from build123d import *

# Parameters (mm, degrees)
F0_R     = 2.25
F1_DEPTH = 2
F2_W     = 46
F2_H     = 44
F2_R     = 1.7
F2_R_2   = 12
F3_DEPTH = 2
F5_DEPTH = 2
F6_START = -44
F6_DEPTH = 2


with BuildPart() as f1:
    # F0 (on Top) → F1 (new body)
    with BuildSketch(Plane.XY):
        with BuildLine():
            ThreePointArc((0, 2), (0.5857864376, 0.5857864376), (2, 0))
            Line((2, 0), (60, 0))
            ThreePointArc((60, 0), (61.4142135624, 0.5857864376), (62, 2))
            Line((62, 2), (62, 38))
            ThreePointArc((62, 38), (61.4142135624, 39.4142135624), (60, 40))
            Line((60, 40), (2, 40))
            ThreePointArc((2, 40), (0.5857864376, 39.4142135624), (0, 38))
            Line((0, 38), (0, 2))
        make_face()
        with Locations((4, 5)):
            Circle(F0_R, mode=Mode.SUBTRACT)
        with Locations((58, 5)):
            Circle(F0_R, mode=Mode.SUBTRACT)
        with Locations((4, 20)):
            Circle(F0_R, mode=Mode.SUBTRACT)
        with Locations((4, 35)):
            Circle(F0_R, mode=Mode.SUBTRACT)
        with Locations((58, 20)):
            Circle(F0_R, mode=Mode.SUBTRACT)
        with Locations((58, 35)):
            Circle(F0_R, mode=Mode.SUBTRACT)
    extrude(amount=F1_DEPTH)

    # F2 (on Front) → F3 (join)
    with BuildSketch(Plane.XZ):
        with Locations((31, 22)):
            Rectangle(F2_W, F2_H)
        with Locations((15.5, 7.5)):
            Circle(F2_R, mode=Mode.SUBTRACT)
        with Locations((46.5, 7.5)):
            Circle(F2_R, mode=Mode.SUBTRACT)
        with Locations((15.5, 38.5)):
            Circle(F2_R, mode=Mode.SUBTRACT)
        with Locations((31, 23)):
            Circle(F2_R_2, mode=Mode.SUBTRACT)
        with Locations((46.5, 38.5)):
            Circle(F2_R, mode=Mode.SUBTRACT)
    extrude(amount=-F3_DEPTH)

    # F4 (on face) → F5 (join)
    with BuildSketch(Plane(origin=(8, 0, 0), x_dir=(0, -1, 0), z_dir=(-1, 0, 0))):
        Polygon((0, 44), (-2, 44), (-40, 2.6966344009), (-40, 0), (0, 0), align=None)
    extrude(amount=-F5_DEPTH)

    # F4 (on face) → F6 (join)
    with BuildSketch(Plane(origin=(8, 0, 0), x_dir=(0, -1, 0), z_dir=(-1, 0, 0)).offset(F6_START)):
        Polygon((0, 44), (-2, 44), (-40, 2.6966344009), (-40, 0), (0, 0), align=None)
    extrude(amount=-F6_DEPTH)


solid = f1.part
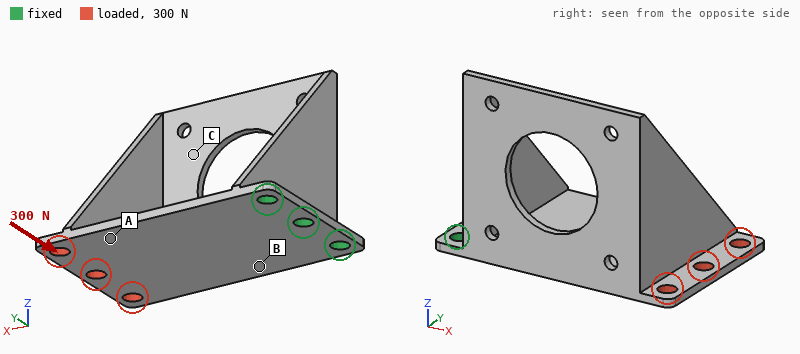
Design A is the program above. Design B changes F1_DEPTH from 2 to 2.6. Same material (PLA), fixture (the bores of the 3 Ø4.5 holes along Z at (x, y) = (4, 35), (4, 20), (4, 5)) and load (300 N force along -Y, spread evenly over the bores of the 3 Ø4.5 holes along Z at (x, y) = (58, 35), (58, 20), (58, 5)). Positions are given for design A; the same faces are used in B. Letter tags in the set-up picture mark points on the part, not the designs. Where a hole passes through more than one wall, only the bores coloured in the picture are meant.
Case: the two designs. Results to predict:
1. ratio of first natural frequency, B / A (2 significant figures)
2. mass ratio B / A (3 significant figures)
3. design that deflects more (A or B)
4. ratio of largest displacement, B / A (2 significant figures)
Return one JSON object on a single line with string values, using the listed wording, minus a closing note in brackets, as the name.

{"ratio of first natural frequency, B / A": "1.3", "mass ratio B / A": "1.12", "design that deflects more": "A", "ratio of largest displacement, B / A": "0.76"}
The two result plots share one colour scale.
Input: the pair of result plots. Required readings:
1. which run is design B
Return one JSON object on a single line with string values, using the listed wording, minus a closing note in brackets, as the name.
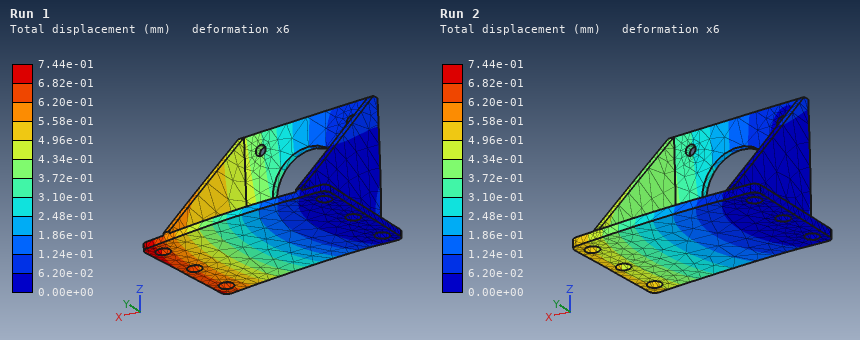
{"which run is design B": "Run 2"}
